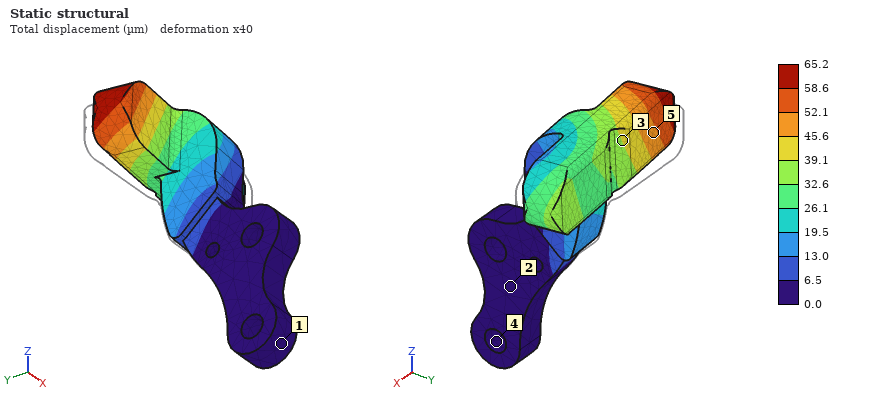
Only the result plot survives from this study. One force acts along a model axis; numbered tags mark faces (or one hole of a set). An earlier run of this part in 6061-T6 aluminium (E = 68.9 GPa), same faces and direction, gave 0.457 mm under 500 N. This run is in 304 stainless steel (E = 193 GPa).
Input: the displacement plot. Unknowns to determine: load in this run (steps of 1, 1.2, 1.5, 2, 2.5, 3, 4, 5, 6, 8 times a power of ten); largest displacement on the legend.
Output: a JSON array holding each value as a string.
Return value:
["200 N", "65.2 µm"]
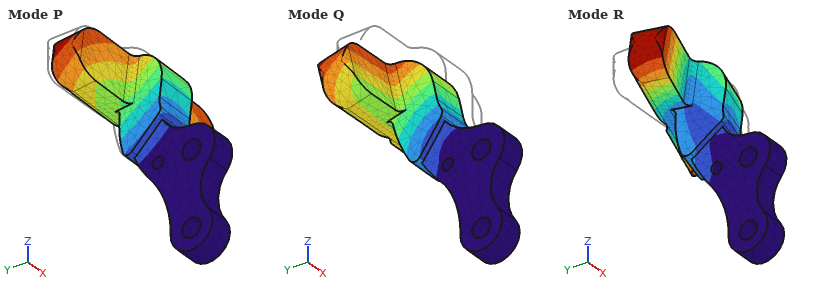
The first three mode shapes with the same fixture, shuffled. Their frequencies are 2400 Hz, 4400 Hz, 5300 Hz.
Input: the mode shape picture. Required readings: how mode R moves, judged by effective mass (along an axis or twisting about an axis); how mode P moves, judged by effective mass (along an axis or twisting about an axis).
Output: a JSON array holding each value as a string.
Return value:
["twisting about Z", "along X"]
